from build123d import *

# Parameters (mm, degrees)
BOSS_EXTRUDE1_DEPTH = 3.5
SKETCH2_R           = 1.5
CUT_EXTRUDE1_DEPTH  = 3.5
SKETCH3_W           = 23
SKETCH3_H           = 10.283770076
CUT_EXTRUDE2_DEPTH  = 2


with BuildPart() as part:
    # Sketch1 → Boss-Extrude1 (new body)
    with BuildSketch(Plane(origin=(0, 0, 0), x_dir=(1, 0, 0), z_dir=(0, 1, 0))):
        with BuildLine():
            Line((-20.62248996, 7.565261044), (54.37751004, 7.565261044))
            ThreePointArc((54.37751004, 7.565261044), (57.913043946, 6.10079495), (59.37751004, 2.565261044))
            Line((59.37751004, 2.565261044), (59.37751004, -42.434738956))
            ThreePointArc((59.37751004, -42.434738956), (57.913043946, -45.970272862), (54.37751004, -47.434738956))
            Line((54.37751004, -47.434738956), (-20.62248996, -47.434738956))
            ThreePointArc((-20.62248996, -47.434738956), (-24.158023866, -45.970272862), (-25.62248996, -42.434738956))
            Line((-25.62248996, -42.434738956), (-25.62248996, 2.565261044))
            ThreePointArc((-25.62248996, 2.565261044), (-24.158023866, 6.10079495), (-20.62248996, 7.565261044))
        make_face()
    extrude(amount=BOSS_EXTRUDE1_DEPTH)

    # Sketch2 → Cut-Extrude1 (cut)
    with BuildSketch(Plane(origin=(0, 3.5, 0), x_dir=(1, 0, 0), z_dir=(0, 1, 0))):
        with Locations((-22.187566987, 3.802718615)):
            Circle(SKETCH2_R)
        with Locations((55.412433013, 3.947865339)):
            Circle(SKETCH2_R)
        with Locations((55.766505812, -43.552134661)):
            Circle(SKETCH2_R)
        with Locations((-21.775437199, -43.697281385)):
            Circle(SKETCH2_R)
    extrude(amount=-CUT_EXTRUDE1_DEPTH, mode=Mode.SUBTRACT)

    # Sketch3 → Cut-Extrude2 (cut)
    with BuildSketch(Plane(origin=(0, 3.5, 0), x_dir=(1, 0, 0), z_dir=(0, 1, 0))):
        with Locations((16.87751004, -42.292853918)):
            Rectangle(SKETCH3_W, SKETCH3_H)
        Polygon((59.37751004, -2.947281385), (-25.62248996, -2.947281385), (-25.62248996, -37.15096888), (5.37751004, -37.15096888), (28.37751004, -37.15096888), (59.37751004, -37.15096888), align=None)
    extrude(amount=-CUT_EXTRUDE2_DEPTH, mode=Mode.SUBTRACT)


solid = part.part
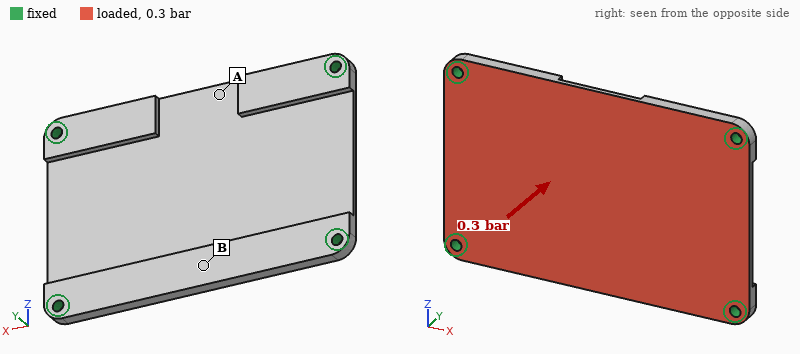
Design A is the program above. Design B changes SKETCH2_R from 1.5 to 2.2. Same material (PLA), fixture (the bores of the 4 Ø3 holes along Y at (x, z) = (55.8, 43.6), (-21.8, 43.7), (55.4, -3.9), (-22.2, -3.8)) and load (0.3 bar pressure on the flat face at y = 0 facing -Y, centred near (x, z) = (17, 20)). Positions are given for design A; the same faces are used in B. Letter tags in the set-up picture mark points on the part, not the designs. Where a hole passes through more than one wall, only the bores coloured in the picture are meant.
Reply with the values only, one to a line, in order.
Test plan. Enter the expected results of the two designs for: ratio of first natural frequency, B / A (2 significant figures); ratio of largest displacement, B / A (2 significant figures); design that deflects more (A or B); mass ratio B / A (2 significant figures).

1.1
0.92
A
0.99
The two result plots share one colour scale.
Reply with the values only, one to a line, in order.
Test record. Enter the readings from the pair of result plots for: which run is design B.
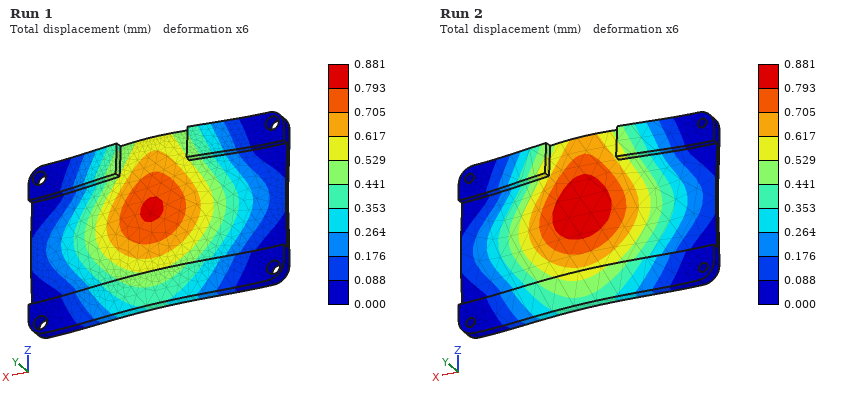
Run 1
